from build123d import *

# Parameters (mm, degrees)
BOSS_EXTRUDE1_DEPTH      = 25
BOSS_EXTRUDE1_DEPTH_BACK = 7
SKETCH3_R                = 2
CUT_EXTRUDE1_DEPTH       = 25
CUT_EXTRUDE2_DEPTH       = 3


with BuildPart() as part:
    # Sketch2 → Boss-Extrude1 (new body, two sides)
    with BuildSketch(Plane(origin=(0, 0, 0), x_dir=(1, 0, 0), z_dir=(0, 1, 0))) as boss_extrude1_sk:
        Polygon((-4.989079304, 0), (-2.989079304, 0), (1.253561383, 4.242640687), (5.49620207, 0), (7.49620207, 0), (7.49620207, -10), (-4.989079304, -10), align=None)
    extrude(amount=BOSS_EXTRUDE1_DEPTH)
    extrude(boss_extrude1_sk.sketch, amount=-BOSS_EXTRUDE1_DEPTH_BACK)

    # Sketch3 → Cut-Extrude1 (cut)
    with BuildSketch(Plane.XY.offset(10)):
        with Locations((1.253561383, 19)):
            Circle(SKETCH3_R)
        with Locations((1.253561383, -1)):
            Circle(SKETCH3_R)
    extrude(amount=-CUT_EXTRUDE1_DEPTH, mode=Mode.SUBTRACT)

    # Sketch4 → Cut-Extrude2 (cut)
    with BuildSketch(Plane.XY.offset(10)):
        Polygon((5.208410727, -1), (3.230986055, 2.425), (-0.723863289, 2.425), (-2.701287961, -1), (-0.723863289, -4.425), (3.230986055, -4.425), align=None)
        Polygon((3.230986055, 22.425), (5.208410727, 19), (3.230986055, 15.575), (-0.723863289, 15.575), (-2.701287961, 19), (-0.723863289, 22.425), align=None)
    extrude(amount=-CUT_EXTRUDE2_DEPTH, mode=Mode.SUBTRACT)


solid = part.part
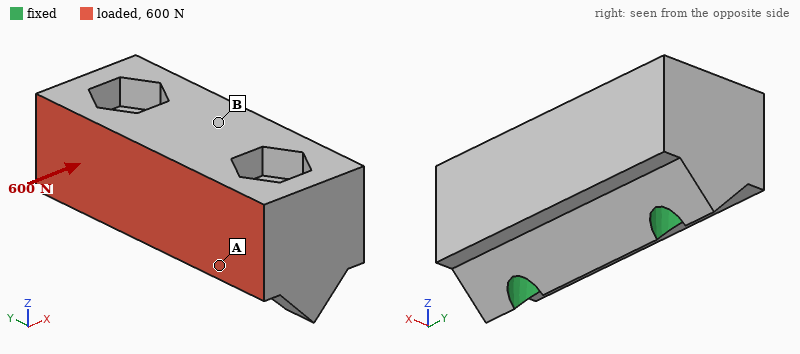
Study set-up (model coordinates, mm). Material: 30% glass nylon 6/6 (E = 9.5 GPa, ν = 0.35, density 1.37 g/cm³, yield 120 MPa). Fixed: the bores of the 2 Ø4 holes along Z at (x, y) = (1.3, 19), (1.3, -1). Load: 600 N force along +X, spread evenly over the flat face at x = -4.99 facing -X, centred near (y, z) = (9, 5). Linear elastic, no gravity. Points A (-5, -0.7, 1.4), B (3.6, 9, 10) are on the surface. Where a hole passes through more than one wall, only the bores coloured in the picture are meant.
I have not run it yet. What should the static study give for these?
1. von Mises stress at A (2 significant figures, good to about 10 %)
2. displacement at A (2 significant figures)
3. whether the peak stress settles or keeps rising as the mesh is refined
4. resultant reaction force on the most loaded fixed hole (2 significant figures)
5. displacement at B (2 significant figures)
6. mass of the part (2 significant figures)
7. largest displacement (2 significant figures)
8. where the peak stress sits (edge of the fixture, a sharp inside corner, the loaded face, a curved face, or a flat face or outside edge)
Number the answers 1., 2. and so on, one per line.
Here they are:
1. 3.0 MPa
2. 1.6 µm
3. keeps rising
4. 300 N
5. 5.1 µm
6. 5.6 g
7. 6.9 µm
8. edge of the fixture
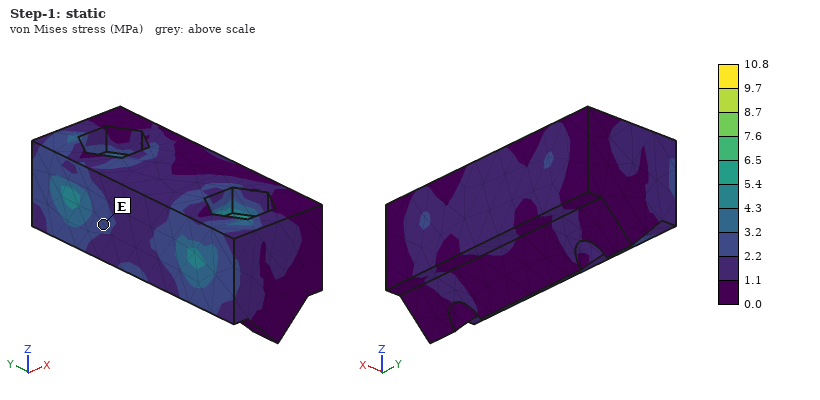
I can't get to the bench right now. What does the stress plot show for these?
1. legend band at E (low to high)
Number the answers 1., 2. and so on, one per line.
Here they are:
1. 2.2 to 3.2 MPa
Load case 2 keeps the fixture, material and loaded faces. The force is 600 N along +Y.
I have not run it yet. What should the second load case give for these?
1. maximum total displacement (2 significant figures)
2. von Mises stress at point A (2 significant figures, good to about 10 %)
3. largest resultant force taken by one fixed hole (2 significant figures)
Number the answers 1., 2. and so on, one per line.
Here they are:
1. 8.9 µm
2. 3.7 MPa
3. 330 N
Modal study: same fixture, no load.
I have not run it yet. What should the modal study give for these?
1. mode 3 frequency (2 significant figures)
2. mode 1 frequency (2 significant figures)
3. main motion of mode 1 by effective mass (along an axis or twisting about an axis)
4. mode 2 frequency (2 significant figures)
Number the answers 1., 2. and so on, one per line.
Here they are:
1. 33 kHz
2. 26 kHz
3. along X
4. 33 kHz
